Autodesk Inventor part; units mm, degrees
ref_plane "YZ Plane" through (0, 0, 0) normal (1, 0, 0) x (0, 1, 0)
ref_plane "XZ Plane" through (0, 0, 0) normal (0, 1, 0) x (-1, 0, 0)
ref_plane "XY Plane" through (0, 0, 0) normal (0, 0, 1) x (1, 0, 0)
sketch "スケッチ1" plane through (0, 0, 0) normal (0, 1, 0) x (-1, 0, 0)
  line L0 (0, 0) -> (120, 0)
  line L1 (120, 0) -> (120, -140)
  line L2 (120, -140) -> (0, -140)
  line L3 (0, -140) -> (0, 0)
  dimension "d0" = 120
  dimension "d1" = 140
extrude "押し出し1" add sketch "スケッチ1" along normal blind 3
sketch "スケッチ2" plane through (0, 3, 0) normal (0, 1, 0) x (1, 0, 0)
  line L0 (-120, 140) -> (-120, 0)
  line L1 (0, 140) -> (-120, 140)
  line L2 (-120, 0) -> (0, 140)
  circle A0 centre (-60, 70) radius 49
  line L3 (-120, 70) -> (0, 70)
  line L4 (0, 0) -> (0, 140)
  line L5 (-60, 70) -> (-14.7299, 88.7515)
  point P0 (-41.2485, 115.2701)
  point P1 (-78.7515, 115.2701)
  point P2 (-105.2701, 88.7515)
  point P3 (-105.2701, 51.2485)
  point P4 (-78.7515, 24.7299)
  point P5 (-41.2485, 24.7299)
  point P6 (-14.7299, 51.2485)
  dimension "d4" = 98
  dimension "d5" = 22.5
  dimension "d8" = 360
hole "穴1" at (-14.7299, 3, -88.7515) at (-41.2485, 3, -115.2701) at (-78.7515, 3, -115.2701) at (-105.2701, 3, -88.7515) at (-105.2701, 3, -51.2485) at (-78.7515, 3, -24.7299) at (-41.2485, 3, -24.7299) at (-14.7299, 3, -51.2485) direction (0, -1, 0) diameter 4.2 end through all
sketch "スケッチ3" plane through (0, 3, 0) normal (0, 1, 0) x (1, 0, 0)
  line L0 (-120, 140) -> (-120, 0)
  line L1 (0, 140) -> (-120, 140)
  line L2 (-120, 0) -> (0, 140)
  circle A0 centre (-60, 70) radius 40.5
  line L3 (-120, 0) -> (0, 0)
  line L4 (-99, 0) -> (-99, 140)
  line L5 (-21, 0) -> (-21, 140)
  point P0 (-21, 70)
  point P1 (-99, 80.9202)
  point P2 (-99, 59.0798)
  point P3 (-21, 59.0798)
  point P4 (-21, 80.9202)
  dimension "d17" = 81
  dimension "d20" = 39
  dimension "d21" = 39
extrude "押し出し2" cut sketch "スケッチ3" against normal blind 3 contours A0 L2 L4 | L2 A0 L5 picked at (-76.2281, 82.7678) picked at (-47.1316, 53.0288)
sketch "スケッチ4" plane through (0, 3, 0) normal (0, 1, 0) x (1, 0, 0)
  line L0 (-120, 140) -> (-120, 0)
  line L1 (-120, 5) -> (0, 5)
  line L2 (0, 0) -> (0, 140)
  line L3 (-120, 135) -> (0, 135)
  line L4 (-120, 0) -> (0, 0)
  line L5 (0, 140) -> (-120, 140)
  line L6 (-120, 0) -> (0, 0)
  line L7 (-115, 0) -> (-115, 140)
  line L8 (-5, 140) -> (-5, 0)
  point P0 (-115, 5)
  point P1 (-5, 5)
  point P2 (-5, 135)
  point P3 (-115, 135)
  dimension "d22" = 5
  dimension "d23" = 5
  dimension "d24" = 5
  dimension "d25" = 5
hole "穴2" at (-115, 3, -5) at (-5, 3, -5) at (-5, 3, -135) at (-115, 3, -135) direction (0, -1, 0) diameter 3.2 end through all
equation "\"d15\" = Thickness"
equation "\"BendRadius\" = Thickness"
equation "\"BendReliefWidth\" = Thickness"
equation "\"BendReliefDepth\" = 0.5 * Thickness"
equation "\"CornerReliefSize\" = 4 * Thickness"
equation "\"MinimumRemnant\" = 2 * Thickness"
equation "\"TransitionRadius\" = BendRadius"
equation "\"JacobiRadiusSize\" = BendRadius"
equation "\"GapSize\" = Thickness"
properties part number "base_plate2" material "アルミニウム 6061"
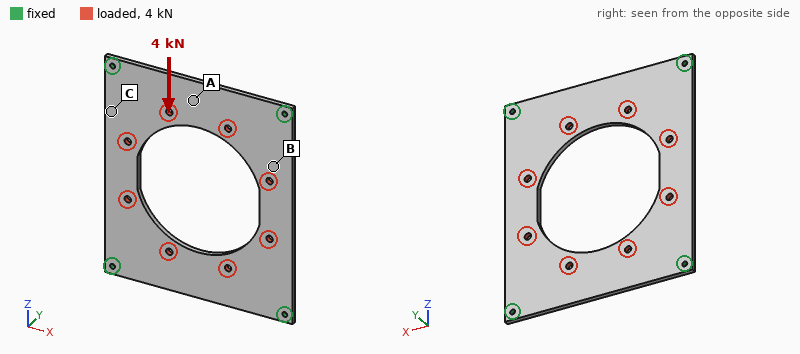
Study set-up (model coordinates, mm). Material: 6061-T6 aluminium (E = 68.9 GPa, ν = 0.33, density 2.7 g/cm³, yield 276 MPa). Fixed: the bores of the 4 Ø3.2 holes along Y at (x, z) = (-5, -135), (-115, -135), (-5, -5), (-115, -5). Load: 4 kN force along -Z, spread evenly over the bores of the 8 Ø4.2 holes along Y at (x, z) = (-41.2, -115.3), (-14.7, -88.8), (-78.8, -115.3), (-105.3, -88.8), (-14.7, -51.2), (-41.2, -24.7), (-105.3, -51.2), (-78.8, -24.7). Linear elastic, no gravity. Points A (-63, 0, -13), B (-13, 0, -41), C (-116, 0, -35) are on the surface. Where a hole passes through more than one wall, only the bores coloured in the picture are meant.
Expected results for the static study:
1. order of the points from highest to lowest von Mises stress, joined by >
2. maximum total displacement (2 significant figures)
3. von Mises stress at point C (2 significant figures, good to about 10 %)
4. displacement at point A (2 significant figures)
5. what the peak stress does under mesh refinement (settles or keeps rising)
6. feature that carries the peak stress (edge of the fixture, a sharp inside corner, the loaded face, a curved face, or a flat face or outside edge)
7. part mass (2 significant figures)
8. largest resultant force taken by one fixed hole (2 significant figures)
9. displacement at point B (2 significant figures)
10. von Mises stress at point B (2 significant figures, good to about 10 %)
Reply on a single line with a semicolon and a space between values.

C > B > A; 23 µm; 16 MPa; 23 µm; keeps rising; edge of the fixture; 94 g; 1.1 kN; 13 µm; 11 MPa
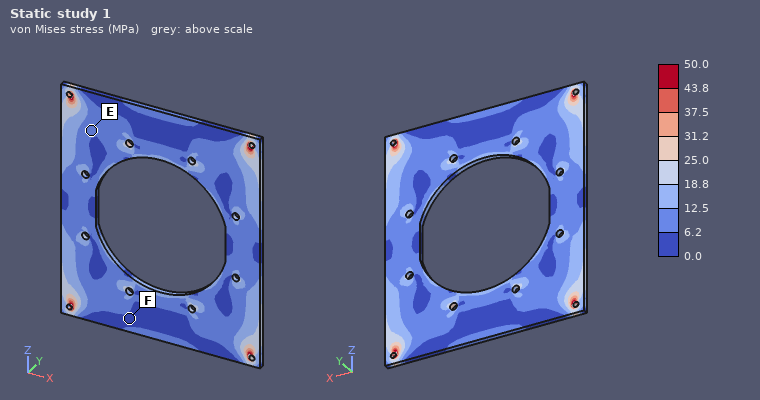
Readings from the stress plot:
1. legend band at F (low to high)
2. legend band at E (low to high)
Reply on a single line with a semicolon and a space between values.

0.0 to 6.2 MPa; 6.2 to 12.5 MPa
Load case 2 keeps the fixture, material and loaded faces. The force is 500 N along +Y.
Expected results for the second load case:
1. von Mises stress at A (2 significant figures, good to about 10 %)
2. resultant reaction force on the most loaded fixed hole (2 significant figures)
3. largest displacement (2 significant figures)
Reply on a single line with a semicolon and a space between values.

23 MPa; 130 N; 0.58 mm
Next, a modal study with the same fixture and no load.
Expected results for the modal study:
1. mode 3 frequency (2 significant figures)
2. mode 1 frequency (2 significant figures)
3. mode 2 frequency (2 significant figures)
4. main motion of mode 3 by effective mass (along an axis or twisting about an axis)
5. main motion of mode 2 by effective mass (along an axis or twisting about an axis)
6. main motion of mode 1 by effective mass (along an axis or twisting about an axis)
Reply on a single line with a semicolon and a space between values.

1200 Hz; 760 Hz; 1000 Hz; twisting about X; twisting about Z; along Y
